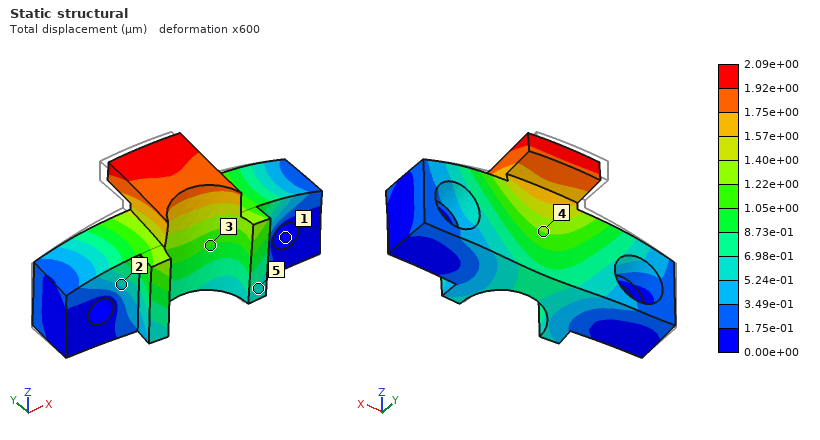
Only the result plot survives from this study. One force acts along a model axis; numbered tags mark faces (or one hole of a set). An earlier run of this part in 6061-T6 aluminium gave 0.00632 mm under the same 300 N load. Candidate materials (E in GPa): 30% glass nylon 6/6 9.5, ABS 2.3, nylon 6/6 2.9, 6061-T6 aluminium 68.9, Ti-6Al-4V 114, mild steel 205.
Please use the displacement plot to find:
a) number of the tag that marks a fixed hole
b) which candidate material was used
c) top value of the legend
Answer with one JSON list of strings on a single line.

["1", "mild steel", "2.09e+00 µm"]
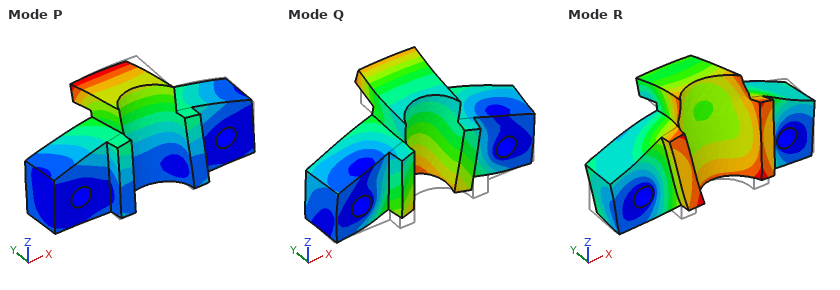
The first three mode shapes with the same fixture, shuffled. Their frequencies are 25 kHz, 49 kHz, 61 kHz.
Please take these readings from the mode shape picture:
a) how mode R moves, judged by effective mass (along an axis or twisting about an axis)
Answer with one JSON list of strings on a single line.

["along Z"]
